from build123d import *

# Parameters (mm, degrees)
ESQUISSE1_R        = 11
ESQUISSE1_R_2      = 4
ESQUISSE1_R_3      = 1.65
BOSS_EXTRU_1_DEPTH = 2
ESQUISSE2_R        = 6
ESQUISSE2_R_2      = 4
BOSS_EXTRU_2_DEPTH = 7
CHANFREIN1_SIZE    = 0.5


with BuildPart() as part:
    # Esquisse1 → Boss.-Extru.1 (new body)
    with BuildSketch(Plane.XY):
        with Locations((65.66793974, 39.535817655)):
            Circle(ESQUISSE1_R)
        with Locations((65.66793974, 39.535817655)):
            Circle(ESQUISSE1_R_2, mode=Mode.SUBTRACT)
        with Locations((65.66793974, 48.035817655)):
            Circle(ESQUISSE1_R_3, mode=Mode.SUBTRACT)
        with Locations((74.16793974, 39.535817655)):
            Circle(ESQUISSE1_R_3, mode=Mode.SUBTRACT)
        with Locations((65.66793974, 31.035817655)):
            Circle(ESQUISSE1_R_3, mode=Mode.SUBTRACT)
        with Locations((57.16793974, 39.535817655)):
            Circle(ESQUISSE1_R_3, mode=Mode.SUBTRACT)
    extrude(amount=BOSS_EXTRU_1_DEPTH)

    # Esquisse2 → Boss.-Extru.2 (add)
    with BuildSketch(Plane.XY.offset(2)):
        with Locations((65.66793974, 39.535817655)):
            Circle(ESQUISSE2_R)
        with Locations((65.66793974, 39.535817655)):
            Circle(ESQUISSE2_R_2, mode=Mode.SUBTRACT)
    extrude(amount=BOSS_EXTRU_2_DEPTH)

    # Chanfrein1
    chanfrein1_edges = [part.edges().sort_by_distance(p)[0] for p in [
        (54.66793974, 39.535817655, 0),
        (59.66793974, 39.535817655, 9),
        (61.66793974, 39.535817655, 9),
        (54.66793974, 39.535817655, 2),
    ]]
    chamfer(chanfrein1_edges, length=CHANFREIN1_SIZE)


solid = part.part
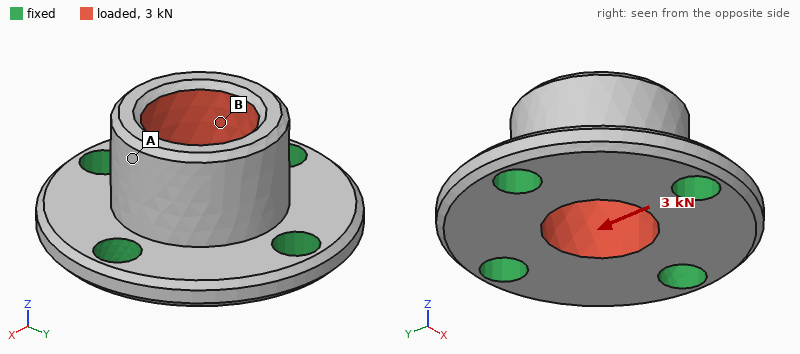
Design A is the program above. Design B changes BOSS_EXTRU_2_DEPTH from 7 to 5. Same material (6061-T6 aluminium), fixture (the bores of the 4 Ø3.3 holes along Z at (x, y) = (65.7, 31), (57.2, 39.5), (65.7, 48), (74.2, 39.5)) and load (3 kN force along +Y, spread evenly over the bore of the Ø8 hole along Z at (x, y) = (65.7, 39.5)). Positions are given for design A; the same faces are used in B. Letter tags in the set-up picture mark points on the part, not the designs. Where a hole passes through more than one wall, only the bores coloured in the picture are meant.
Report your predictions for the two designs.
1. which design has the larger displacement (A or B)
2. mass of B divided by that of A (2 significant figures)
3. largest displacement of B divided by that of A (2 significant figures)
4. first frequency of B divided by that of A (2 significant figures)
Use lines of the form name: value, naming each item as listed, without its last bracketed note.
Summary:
which design has the larger displacement: A
mass of B divided by that of A: 0.88
largest displacement of B divided by that of A: 0.64
first frequency of B divided by that of A: 1.3
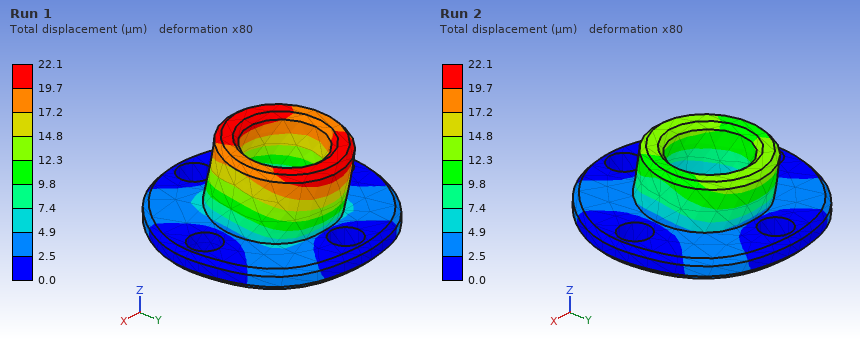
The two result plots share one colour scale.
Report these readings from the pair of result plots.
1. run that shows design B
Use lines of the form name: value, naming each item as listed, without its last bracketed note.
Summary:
run that shows design B: Run 2
